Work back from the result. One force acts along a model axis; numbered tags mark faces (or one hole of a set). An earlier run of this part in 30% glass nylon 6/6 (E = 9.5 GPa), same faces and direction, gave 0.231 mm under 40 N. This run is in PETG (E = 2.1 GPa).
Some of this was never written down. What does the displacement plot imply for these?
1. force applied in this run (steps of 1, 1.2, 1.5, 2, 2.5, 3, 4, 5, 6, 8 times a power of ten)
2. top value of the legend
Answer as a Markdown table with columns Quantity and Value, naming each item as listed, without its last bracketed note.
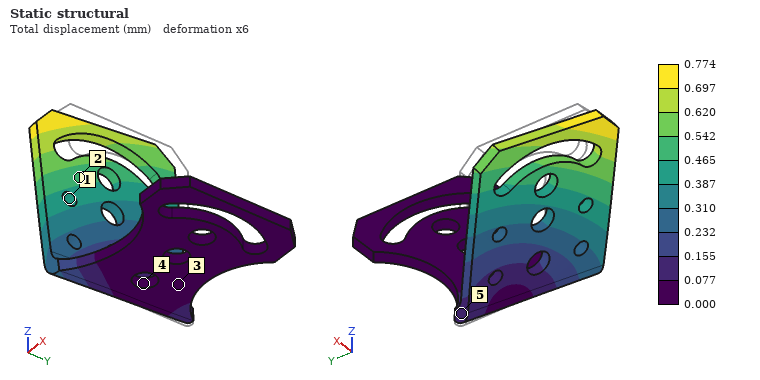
| Quantity | Value |
|---|---|
| force applied in this run | 30 N |
| top value of the legend | 0.774 mm |
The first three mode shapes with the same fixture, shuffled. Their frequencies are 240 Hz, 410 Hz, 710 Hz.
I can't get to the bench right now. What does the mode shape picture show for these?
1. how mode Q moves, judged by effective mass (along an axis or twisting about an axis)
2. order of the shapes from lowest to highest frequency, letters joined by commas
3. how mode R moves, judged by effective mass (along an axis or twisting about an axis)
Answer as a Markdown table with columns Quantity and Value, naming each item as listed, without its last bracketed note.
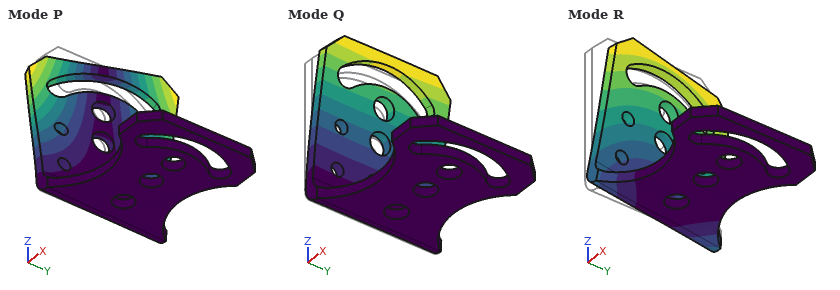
| Quantity | Value |
|---|---|
| how mode Q moves, judged by effective mass | along X |
| order of the shapes from lowest to highest frequency, letters joined by commas | Q, R, P |
| how mode R moves, judged by effective mass | along Y |
